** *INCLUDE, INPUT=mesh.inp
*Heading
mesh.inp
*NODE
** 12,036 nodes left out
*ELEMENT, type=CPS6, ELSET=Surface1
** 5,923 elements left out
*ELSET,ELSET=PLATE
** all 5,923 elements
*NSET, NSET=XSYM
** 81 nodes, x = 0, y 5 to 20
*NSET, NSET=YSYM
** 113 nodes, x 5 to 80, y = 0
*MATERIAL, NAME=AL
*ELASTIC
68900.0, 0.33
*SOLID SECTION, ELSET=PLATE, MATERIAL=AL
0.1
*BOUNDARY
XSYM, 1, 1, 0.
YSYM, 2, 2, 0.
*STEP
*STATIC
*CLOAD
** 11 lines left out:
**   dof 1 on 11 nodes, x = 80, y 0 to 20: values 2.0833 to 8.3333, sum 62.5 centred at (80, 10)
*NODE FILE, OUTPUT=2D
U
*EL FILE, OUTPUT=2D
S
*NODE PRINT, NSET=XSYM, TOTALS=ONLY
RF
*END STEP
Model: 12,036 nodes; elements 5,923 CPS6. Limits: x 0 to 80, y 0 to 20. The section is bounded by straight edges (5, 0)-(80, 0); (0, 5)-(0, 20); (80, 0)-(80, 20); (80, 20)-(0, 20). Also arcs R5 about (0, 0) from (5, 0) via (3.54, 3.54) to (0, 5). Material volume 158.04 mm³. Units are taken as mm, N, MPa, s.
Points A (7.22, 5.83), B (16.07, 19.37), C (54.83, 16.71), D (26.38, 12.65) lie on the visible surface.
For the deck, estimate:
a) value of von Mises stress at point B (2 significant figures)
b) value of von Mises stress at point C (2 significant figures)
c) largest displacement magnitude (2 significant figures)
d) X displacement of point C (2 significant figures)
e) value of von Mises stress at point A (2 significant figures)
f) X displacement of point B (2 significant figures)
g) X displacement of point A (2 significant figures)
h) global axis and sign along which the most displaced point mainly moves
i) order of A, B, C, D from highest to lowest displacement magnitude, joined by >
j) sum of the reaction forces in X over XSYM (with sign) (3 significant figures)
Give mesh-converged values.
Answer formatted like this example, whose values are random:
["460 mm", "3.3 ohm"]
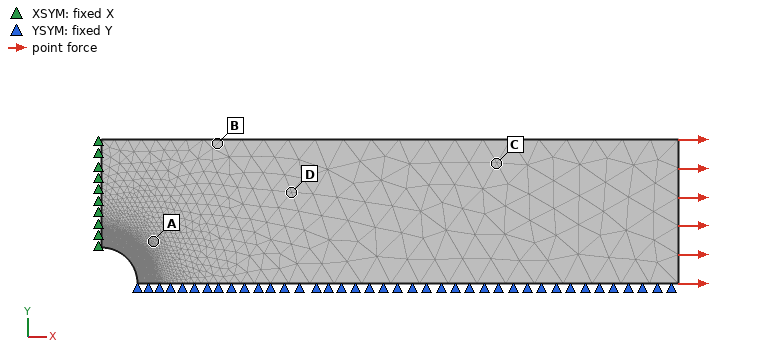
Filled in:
["37 MPa", "31 MPa", "0.039 mm", "0.026 mm", "41 MPa", "0.0079 mm", "0.0053 mm", "+X", "C > D > B > A", "-62.5 N"]
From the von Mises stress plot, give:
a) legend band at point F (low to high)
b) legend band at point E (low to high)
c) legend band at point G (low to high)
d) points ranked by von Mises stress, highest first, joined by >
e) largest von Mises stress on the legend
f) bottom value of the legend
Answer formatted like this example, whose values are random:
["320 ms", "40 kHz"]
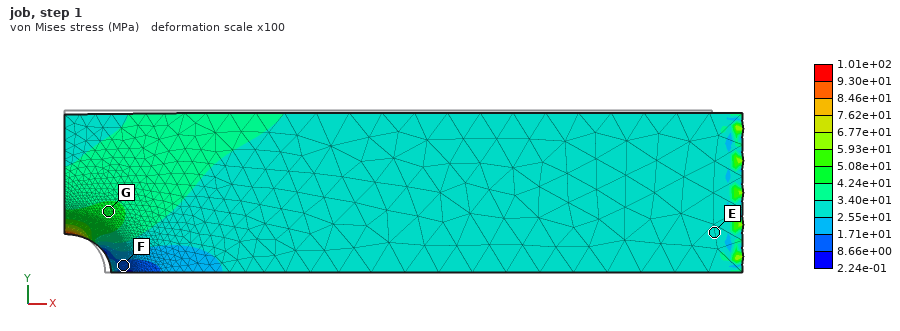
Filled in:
["8.66e+00 to 1.71e+01 MPa", "2.55e+01 to 3.40e+01 MPa", "4.24e+01 to 5.08e+01 MPa", "G > E > F", "1.01e+02 MPa", "2.24e-01 MPa"]
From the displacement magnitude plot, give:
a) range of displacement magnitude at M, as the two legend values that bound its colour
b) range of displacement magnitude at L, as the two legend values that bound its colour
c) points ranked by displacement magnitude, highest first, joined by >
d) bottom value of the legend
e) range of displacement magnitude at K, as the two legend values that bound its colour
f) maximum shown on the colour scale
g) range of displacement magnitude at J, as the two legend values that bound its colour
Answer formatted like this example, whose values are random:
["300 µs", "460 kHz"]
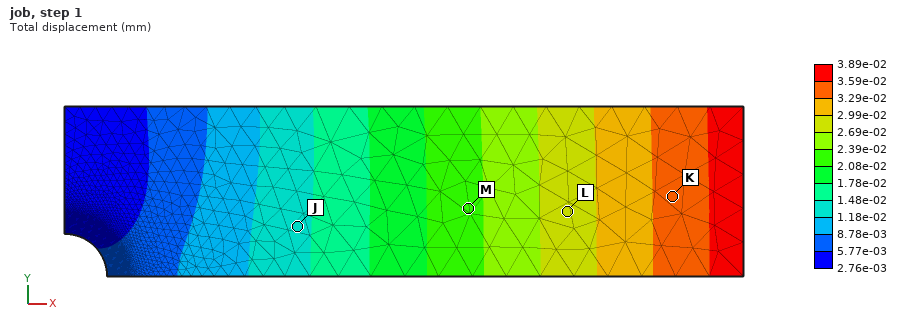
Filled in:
["2.08e-02 to 2.39e-02 mm", "2.69e-02 to 2.99e-02 mm", "K > L > M > J", "2.76e-03 mm", "3.29e-02 to 3.59e-02 mm", "3.89e-02 mm", "1.18e-02 to 1.48e-02 mm"]
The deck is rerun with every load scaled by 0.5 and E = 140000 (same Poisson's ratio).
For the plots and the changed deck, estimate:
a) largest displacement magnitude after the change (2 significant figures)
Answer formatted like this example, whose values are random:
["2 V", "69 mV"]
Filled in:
["0.0096 mm"]
